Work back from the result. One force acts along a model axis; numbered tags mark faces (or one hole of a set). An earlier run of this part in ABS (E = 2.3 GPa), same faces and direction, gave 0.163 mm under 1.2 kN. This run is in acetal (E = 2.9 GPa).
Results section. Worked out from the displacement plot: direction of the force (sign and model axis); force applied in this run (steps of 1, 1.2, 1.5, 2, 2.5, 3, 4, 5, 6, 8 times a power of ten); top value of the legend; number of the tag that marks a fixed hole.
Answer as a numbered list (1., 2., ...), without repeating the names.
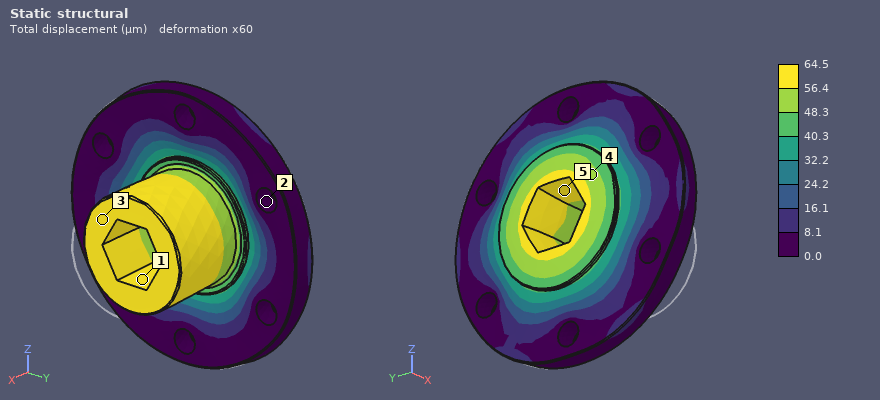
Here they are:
1. -X
2. 600 N
3. 64.5 µm
4. 2
